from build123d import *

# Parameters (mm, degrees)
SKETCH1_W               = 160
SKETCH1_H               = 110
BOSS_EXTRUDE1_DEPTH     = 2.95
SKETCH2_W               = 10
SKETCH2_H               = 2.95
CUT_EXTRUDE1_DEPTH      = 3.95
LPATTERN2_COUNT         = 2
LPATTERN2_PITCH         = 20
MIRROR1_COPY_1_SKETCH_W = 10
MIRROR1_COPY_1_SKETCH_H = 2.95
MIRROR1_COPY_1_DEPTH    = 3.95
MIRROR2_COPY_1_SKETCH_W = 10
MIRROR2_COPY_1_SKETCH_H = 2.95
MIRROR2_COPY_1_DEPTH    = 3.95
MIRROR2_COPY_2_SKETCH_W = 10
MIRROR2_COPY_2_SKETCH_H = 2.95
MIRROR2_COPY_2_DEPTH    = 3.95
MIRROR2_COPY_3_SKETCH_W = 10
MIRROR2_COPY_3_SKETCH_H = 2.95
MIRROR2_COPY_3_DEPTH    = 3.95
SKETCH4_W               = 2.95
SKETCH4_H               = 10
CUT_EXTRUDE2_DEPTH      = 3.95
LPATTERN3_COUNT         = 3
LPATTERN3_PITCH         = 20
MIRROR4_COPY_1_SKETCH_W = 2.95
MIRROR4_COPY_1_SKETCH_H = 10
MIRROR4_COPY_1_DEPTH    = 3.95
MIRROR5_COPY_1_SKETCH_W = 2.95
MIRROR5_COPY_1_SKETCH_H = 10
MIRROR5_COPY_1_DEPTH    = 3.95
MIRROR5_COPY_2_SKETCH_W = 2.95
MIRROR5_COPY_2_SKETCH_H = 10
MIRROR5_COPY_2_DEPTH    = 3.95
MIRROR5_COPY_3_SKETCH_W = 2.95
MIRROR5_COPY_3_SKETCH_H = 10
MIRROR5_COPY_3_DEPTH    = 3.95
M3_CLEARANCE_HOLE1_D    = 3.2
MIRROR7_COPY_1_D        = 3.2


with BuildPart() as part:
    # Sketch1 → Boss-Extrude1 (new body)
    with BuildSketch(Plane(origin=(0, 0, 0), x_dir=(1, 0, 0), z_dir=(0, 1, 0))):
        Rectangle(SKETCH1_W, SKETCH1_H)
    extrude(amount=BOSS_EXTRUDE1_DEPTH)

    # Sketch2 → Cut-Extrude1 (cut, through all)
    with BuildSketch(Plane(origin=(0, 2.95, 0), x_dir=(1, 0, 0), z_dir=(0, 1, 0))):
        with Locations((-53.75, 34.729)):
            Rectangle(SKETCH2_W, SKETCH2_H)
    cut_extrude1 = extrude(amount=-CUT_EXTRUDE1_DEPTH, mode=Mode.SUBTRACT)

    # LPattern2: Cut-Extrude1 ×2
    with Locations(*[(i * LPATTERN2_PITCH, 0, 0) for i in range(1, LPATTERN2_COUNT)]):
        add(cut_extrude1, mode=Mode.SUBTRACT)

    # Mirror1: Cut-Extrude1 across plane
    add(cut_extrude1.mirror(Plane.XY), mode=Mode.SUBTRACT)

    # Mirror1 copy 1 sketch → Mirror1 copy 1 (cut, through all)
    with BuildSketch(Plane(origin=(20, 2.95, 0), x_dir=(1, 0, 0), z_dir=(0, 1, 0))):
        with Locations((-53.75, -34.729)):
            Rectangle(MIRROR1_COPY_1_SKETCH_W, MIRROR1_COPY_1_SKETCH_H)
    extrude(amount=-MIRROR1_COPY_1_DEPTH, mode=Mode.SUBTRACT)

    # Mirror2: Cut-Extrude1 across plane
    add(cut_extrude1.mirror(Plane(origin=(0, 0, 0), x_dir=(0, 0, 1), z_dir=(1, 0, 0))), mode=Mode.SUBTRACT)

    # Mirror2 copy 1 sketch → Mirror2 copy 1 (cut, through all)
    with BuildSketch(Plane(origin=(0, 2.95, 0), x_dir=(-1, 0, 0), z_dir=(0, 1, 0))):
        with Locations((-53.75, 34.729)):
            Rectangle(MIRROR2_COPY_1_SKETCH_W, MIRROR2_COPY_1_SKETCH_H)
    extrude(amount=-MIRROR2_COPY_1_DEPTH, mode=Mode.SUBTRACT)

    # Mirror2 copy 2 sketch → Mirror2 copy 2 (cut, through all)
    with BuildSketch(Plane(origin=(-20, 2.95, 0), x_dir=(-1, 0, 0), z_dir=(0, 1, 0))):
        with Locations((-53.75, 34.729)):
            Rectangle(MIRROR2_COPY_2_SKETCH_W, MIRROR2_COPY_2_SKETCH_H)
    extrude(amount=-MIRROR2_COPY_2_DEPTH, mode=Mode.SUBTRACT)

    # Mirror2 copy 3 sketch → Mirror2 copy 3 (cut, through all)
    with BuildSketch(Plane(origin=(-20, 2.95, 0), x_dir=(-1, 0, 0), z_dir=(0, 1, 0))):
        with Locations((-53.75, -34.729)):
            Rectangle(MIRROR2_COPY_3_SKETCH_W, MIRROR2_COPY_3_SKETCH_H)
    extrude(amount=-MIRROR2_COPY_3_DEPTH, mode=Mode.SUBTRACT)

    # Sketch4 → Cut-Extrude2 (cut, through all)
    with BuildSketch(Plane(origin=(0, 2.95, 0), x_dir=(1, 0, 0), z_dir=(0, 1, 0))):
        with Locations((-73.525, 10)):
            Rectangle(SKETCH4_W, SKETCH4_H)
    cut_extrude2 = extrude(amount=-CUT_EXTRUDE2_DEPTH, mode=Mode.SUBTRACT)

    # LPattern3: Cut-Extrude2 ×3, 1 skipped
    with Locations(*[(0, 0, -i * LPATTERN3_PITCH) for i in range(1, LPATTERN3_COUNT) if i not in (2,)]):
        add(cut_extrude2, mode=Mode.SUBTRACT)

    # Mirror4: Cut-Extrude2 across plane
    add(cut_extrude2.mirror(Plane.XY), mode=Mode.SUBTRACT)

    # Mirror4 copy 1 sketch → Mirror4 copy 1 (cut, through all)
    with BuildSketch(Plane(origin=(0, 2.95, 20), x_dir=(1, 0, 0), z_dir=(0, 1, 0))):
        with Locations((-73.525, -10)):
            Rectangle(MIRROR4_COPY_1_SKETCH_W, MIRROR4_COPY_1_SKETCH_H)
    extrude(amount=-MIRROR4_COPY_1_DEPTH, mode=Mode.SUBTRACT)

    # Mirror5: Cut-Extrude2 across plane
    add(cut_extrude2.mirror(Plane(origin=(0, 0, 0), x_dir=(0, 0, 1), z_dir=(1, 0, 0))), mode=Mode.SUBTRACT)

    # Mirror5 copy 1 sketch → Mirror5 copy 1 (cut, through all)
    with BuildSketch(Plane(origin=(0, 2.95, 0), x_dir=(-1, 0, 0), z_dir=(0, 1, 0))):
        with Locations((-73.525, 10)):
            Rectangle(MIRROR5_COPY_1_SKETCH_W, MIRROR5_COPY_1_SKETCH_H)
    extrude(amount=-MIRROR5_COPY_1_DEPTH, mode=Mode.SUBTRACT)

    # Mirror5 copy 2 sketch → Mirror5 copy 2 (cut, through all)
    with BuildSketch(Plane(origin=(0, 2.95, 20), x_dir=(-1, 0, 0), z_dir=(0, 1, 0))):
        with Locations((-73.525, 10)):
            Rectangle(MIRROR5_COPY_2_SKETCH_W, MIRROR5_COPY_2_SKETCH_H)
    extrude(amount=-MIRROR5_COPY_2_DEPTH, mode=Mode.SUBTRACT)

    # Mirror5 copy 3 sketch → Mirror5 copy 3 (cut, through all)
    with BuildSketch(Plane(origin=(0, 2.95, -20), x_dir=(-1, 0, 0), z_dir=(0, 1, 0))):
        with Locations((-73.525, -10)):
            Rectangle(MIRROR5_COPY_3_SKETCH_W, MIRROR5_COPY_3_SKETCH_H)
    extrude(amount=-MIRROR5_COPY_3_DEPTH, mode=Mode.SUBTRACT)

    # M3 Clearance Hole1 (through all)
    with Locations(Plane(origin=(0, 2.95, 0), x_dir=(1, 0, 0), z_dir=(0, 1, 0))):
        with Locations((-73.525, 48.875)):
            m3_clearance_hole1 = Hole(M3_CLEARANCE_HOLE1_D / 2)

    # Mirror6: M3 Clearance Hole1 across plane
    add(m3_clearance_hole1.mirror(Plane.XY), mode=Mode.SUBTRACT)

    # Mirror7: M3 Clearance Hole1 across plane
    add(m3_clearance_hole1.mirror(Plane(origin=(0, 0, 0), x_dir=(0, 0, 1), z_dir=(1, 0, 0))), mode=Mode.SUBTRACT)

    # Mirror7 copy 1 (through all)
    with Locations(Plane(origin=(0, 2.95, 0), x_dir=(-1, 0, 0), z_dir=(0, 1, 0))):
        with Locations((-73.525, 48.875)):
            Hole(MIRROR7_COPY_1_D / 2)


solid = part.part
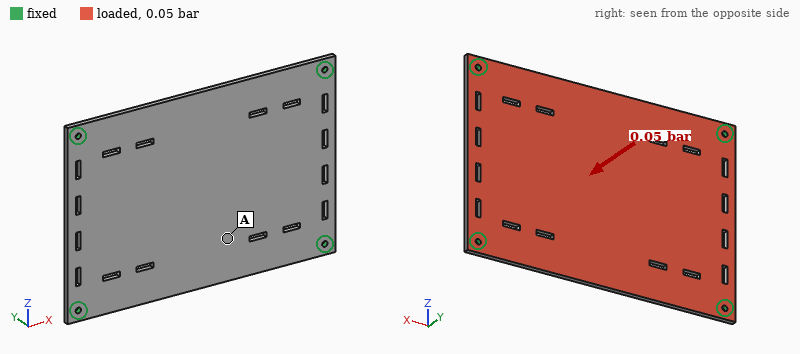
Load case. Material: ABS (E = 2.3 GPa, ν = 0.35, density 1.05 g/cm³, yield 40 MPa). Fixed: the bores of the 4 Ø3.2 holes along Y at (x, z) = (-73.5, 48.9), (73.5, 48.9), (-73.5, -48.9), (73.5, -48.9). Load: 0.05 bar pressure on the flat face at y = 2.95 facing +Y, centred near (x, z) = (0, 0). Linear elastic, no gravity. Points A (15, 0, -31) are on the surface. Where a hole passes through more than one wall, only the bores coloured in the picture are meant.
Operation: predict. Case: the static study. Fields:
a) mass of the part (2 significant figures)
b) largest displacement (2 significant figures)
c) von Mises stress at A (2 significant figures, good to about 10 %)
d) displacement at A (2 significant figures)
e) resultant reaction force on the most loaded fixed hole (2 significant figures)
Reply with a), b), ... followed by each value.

a) 53 g
b) 2.2 mm
c) 3.5 MPa
d) 2.0 mm
e) 21 N
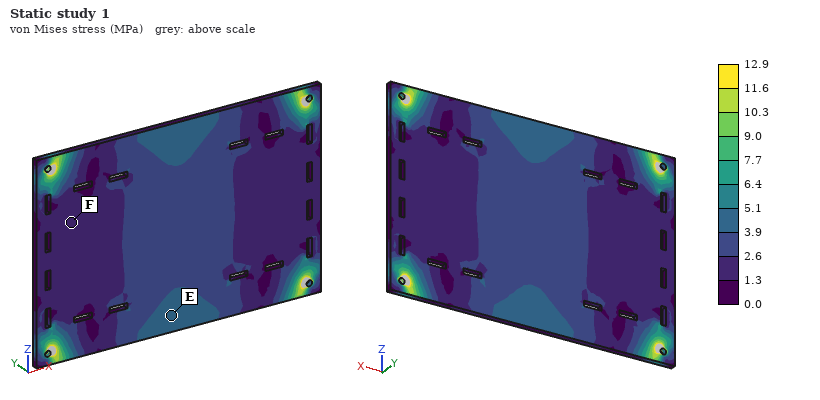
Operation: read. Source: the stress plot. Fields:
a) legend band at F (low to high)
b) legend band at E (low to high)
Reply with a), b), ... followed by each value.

a) 1.3 to 2.6 MPa
b) 3.9 to 5.1 MPa
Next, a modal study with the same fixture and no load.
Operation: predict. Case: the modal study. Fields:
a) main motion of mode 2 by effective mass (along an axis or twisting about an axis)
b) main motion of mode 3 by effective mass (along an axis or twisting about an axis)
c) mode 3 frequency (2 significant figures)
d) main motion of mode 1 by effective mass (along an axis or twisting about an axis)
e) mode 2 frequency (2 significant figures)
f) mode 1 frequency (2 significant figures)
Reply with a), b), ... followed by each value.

a) twisting about X
b) twisting about Z
c) 390 Hz
d) along Y
e) 260 Hz
f) 160 Hz
